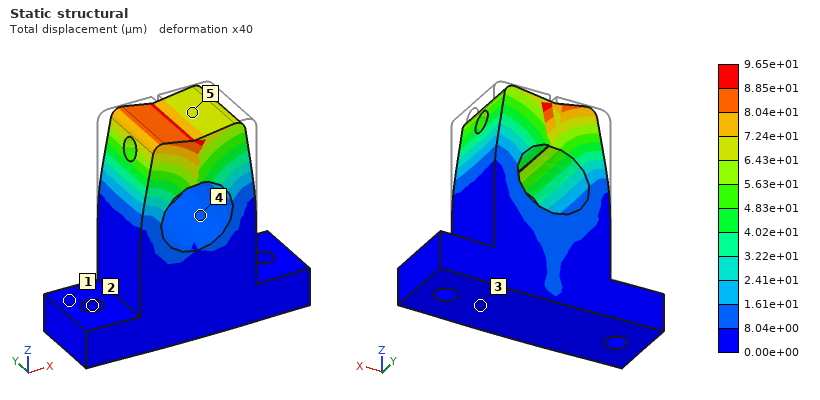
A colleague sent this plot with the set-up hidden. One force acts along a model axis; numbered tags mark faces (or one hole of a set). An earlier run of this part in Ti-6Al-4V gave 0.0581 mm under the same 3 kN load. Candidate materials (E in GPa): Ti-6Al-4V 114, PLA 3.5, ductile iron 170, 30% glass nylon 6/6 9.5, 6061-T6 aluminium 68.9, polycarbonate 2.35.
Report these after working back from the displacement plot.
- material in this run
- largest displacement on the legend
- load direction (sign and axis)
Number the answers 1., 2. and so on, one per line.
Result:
1. 6061-T6 aluminium
2. 9.65e+01 µm
3. -Z
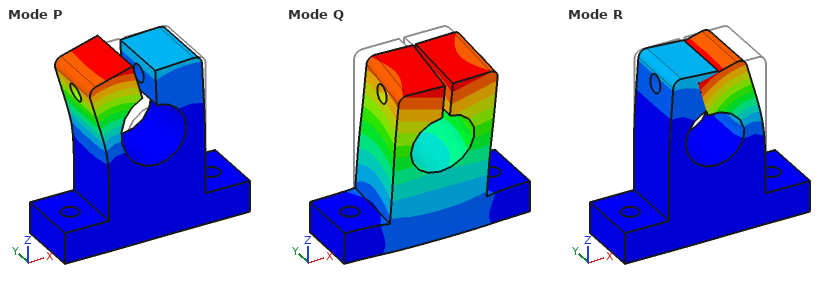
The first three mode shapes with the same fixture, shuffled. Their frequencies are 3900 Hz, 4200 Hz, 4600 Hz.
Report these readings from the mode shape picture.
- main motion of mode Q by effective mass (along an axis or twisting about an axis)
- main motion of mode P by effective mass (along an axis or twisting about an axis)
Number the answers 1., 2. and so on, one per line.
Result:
1. along Y
2. along X
